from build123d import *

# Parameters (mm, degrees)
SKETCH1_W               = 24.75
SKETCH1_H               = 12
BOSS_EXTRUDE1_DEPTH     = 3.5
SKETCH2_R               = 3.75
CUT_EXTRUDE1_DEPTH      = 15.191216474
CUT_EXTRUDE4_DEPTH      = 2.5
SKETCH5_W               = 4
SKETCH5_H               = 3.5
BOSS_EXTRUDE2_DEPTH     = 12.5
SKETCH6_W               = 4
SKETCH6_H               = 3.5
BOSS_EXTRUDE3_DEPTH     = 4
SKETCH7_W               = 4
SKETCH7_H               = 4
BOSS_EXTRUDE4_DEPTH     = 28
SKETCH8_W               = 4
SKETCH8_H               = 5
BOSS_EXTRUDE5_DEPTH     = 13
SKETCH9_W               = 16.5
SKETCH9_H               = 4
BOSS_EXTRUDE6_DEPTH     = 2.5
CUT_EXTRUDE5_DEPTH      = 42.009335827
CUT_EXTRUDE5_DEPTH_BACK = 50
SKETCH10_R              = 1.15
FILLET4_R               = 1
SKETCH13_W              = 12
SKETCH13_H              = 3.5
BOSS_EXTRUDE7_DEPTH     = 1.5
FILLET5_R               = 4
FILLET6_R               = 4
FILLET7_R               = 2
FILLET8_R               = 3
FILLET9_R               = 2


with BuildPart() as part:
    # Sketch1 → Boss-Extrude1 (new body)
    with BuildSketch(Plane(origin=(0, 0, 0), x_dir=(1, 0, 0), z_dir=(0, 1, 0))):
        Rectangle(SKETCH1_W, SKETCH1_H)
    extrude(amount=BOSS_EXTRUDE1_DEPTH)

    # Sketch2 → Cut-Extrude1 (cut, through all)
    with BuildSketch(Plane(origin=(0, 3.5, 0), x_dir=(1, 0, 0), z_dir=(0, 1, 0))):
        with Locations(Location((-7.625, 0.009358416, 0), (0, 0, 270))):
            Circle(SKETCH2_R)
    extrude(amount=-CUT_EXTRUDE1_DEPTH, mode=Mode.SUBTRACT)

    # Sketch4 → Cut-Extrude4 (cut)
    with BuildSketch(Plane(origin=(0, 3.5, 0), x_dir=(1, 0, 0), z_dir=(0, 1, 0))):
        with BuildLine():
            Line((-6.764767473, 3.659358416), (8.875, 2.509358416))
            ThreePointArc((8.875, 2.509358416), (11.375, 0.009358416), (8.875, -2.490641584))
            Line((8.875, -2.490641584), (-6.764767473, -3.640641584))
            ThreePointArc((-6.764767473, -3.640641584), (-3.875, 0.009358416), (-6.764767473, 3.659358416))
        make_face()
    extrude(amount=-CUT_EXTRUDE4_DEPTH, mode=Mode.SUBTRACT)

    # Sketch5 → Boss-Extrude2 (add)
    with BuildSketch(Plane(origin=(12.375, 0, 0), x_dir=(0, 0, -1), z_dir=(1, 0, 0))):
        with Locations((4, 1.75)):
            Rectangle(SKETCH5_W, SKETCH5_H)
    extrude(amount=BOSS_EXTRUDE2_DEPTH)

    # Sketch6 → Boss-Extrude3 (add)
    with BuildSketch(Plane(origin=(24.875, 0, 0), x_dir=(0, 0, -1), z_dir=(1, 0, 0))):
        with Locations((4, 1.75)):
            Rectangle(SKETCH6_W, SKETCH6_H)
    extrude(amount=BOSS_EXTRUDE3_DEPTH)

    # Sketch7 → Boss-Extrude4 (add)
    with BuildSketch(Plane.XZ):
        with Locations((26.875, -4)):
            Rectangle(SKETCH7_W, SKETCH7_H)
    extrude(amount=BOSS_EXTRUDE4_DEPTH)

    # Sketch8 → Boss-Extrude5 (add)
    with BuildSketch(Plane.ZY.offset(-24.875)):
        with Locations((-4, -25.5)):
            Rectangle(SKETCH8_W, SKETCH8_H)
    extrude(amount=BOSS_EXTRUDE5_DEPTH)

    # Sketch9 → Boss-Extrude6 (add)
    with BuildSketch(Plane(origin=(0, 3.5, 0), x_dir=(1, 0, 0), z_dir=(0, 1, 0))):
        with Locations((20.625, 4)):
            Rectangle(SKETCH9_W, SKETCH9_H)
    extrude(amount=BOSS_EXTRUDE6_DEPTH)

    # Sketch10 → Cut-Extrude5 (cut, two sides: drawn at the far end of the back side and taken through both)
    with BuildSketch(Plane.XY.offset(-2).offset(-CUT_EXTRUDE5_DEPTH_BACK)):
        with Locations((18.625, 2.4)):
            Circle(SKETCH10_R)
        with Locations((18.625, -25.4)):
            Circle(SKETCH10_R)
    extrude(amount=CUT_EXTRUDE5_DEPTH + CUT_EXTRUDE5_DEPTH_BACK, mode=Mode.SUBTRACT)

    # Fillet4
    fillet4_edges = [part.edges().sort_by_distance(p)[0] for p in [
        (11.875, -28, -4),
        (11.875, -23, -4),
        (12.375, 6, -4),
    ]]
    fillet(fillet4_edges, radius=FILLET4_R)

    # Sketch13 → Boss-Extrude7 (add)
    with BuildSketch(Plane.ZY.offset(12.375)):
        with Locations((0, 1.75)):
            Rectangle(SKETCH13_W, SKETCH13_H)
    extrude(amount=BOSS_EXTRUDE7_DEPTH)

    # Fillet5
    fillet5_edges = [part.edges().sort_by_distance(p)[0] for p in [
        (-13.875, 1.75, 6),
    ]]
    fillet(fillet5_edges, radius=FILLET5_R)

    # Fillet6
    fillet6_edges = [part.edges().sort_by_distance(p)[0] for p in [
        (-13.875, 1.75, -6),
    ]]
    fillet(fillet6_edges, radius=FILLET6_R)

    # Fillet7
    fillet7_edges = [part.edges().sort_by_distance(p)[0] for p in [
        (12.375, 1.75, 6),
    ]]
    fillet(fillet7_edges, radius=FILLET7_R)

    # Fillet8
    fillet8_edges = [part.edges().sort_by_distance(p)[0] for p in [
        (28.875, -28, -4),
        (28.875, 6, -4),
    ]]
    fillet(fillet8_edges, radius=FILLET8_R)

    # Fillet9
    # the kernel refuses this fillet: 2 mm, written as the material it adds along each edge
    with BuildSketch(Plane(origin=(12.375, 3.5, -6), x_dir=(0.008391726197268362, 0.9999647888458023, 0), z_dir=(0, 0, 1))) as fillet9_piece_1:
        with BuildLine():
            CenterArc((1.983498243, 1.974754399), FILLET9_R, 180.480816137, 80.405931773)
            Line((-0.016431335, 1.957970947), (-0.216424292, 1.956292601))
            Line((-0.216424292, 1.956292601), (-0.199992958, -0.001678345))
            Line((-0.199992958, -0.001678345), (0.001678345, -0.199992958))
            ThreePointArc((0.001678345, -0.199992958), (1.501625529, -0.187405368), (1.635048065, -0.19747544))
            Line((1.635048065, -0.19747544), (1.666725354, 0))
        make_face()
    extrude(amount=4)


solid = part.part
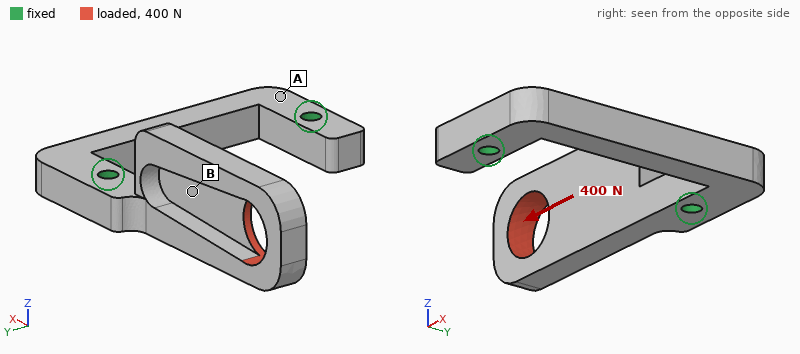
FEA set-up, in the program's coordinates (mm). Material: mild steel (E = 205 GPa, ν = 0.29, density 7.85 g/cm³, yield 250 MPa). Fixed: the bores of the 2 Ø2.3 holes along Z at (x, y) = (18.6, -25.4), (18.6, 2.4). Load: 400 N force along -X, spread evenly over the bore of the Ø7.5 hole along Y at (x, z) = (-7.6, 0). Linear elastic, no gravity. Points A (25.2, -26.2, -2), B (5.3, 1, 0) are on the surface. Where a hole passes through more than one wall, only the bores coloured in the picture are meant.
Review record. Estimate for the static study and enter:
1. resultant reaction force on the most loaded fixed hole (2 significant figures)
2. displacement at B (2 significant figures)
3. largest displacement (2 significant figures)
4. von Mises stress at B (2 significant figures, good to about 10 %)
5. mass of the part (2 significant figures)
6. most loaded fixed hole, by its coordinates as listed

400 N
27 µm
82 µm
44 MPa
14 g
(18.6, 2.4)
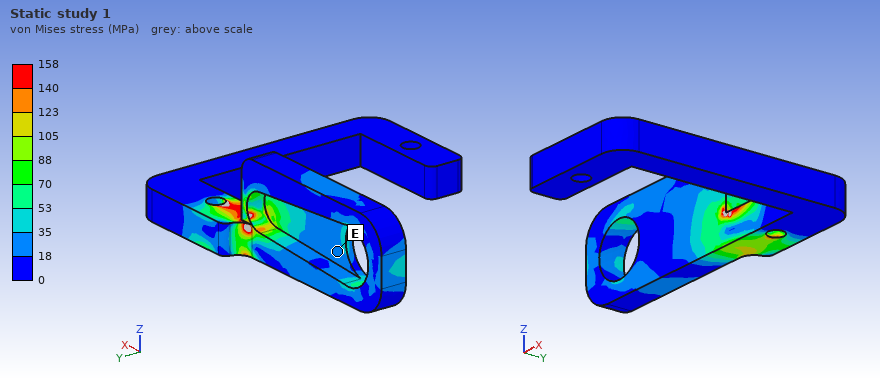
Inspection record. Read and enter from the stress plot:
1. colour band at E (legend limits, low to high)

18 to 35 MPa
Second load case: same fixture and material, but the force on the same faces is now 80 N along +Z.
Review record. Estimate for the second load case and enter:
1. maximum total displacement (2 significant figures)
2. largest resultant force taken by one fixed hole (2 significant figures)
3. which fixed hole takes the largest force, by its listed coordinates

100 µm
80 N
(18.6, 2.4)
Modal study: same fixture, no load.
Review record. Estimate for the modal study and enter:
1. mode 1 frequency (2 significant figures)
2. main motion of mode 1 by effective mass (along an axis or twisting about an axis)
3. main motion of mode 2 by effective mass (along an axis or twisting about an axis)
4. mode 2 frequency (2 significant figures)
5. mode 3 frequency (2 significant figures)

2600 Hz
along Y
along Z
3000 Hz
7600 Hz
